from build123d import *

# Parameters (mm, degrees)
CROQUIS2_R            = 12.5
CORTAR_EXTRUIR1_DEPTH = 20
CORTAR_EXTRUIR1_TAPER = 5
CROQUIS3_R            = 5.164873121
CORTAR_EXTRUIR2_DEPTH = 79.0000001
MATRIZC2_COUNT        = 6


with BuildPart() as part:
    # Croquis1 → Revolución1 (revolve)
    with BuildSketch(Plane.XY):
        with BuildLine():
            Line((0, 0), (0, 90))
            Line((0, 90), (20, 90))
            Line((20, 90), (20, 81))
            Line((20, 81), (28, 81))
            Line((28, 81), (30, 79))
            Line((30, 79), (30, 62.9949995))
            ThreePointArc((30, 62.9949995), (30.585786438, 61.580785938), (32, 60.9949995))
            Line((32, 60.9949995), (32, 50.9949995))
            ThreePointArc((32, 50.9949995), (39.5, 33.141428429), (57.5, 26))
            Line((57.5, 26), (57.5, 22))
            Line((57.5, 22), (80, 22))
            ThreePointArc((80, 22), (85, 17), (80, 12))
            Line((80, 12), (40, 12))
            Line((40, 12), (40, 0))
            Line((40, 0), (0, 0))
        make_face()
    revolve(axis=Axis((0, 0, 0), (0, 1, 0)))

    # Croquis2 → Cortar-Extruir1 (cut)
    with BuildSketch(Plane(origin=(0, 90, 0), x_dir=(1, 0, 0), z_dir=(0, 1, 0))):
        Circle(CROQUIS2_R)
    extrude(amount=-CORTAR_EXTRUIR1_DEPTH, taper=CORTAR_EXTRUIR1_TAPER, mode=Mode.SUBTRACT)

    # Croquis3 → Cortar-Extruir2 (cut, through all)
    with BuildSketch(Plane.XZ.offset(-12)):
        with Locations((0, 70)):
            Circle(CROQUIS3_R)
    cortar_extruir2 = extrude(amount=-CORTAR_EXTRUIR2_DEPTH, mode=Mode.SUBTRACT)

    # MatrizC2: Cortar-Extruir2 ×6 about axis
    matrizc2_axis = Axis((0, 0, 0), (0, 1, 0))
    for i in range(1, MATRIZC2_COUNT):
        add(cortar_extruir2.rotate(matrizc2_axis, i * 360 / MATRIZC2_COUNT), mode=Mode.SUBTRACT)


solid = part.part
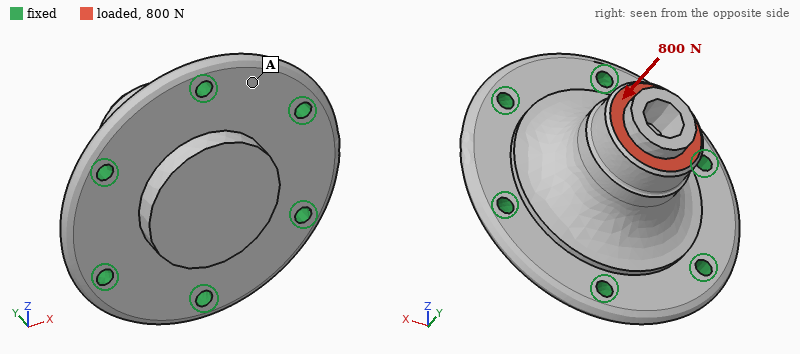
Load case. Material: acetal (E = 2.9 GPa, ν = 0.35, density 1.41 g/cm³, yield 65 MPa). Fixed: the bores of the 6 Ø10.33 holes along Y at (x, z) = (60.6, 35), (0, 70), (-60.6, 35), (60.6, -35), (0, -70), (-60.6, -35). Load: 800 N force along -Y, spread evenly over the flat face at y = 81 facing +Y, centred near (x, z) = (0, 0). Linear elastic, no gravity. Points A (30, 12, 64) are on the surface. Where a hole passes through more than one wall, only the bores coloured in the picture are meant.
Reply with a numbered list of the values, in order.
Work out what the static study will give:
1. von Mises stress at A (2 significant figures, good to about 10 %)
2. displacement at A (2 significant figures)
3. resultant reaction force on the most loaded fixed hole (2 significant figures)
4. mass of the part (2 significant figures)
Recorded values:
1. 0.34 MPa
2. 7.9 µm
3. 150 N
4. 740 g
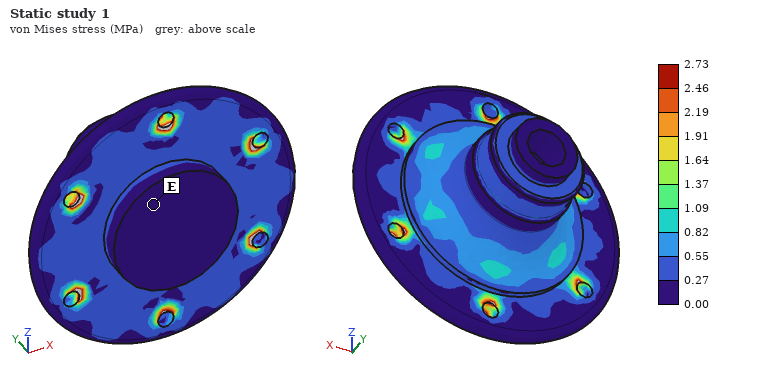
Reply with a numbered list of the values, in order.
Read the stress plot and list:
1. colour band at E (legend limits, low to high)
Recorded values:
1. 0.00 to 0.27 MPa
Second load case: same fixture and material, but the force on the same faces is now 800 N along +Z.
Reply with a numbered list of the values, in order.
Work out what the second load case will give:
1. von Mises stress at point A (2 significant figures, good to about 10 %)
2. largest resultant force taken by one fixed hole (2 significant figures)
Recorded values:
1. 0.69 MPa
2. 360 N
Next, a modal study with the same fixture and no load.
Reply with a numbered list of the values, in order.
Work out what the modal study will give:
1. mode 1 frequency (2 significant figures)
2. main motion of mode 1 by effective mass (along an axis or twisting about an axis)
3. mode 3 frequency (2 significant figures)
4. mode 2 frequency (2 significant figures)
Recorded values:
1. 1300 Hz
2. along Y
3. 1500 Hz
4. 1500 Hz
